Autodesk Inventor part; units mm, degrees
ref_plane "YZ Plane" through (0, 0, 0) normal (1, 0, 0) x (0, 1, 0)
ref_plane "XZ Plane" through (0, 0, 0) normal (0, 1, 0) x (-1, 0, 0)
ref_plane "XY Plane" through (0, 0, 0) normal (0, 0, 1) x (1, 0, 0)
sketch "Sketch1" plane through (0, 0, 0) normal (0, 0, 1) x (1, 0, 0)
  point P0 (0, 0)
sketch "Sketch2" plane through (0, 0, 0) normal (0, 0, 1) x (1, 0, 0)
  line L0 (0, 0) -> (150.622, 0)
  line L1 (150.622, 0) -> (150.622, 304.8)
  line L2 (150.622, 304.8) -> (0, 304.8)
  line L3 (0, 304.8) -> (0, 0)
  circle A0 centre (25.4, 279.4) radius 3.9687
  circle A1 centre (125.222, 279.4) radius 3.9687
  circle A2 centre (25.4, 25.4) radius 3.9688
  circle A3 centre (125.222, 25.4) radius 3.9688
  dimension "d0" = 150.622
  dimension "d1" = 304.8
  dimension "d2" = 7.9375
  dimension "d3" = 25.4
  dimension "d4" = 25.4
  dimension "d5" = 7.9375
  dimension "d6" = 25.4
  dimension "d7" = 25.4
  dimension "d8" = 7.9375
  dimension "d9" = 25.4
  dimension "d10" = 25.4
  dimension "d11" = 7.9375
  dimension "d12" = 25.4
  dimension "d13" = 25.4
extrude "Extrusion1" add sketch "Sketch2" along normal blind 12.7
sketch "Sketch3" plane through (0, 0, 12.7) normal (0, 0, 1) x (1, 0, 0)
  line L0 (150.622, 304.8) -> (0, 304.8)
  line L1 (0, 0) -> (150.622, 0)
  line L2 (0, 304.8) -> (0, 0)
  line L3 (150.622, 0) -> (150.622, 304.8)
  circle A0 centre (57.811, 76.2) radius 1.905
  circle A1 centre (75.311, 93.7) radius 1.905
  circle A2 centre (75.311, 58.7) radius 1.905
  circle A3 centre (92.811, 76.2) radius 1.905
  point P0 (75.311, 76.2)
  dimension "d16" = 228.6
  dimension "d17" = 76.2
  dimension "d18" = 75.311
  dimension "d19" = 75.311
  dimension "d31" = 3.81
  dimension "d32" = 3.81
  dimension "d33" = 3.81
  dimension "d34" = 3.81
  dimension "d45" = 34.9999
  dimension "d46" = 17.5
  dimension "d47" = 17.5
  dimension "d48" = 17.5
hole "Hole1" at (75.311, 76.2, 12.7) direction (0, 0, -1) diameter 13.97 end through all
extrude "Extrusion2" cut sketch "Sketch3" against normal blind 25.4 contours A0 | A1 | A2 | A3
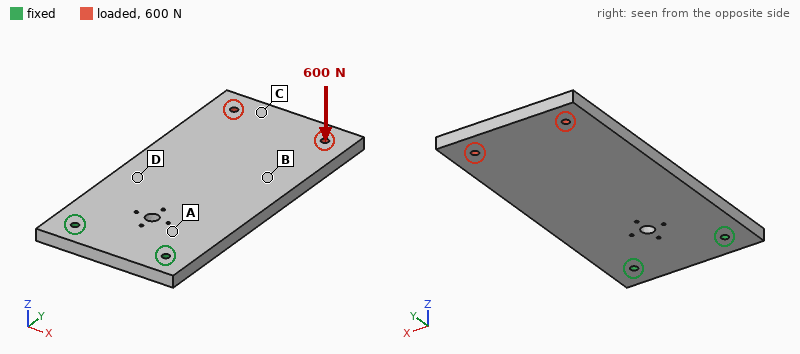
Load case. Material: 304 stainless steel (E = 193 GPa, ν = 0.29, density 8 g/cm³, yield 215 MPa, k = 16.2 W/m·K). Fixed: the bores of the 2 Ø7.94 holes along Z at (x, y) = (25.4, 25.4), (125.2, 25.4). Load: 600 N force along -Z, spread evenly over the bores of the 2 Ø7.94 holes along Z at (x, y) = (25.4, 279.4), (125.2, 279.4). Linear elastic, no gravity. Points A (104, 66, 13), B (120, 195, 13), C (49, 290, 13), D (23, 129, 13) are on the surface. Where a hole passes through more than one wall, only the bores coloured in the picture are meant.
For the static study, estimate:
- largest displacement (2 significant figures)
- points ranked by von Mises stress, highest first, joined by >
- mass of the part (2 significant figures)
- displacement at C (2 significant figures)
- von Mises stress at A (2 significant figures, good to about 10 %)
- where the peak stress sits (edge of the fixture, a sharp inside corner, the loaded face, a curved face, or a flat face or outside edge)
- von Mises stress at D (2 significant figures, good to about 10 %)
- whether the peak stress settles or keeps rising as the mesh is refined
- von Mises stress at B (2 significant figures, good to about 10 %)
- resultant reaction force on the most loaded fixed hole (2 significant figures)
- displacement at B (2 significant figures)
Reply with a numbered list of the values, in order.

1. 0.85 mm
2. A > D > B > C
3. 4.6 kg
4. 0.79 mm
5. 31 MPa
6. edge of the fixture
7. 22 MPa
8. keeps rising
9. 13 MPa
10. 300 N
11. 0.40 mm
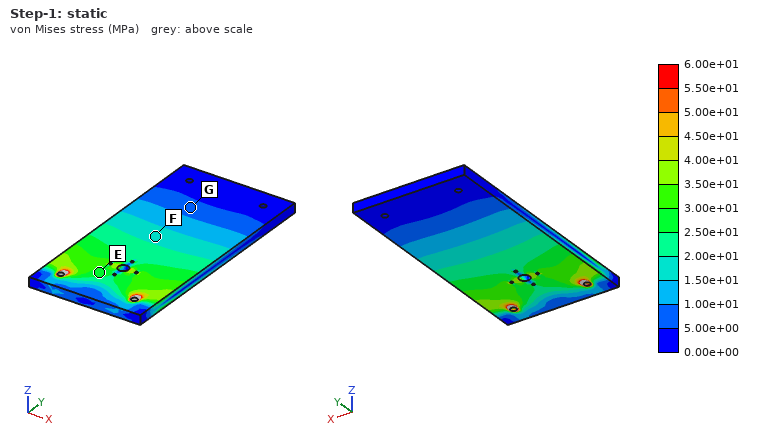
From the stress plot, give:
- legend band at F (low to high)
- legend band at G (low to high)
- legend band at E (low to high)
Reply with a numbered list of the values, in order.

1. 1.50e+01 to 2.00e+01 MPa
2. 5.00e+00 to 1.00e+01 MPa
3. 2.50e+01 to 3.00e+01 MPa
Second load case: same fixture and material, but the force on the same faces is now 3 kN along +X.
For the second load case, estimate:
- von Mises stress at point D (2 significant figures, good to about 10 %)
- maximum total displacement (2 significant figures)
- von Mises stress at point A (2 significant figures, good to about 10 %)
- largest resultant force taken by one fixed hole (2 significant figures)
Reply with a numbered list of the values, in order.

1. 6.8 MPa
2. 42 µm
3. 7.6 MPa
4. 7.6 kN
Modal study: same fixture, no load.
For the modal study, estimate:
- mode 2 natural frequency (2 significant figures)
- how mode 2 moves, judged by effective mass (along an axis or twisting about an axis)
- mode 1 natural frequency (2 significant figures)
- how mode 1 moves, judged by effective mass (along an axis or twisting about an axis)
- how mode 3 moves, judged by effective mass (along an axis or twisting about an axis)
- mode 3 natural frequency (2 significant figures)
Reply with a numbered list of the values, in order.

1. 510 Hz
2. twisting about Y
3. 120 Hz
4. along Z
5. along Z
6. 770 Hz
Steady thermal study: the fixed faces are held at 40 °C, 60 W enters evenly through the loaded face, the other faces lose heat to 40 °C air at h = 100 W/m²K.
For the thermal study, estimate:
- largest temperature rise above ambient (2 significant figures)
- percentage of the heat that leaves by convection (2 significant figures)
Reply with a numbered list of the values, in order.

1. 64 K
2. 100 %
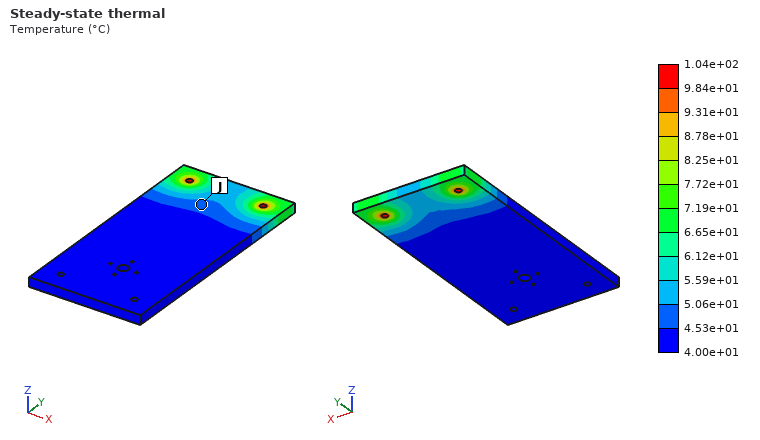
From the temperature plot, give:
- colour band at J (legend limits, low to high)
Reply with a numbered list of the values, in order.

1. 4.53e+01 to 5.06e+01 °C
